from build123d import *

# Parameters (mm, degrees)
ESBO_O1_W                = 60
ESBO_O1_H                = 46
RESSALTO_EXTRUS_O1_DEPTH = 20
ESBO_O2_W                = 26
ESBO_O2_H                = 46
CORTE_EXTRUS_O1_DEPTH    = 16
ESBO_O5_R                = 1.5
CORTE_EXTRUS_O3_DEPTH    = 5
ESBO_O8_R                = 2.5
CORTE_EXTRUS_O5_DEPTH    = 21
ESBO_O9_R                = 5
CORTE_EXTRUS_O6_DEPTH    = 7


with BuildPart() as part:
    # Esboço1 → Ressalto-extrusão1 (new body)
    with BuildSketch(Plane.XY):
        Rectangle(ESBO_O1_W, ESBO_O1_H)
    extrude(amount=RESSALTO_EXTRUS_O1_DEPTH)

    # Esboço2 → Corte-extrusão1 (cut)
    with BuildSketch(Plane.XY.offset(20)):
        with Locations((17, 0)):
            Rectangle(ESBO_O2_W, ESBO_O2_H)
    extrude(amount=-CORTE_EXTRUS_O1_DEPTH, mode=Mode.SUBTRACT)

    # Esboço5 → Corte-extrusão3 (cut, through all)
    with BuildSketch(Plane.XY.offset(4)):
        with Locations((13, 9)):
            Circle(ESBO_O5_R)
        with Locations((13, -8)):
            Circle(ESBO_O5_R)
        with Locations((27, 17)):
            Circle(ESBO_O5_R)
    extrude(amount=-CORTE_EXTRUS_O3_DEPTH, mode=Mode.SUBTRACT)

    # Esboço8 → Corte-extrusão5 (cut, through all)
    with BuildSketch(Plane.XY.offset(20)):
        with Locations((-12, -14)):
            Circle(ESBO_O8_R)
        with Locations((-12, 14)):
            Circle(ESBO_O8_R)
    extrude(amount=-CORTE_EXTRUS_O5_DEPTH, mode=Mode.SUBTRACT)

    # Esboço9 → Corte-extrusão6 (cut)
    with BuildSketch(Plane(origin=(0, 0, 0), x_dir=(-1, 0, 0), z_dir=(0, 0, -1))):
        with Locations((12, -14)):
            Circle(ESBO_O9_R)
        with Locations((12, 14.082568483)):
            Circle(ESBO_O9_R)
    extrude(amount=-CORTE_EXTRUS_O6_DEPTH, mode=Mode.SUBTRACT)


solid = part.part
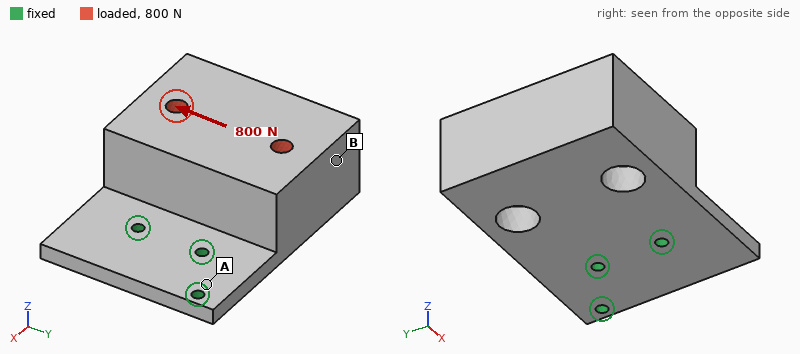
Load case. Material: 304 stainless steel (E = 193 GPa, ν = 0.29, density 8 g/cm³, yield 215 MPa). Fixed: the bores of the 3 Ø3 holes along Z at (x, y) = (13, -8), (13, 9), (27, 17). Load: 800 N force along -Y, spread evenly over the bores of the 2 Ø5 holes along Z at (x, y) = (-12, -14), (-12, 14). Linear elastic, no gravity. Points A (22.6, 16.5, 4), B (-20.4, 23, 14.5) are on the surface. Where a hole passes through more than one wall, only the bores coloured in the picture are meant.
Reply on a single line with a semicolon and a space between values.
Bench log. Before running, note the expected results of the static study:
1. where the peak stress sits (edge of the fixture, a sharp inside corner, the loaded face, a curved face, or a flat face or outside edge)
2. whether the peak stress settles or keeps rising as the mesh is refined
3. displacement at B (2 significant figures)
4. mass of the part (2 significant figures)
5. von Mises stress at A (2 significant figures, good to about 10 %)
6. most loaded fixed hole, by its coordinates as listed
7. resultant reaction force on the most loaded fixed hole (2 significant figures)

edge of the fixture; keeps rising; 11 µm; 270 g; 9.7 MPa; (13, -8); 1.0 kN
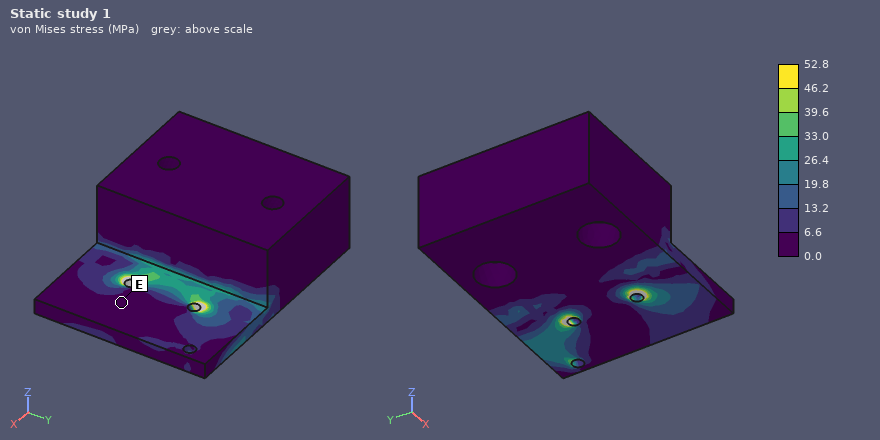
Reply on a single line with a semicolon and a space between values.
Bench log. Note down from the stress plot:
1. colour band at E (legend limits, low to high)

0.0 to 6.6 MPa
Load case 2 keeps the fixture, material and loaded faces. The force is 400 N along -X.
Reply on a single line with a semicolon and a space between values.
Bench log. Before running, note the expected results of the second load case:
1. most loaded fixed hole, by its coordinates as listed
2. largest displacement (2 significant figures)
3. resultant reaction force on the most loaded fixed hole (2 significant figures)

(13, -8); 49 µm; 220 N
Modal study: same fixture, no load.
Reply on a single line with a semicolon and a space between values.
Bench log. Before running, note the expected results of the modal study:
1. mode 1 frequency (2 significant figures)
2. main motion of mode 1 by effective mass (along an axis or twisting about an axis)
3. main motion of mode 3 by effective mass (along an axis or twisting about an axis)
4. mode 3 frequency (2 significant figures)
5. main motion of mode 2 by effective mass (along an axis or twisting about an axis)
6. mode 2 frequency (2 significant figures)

800 Hz; along Z; along Y; 4800 Hz; along Y; 3000 Hz
